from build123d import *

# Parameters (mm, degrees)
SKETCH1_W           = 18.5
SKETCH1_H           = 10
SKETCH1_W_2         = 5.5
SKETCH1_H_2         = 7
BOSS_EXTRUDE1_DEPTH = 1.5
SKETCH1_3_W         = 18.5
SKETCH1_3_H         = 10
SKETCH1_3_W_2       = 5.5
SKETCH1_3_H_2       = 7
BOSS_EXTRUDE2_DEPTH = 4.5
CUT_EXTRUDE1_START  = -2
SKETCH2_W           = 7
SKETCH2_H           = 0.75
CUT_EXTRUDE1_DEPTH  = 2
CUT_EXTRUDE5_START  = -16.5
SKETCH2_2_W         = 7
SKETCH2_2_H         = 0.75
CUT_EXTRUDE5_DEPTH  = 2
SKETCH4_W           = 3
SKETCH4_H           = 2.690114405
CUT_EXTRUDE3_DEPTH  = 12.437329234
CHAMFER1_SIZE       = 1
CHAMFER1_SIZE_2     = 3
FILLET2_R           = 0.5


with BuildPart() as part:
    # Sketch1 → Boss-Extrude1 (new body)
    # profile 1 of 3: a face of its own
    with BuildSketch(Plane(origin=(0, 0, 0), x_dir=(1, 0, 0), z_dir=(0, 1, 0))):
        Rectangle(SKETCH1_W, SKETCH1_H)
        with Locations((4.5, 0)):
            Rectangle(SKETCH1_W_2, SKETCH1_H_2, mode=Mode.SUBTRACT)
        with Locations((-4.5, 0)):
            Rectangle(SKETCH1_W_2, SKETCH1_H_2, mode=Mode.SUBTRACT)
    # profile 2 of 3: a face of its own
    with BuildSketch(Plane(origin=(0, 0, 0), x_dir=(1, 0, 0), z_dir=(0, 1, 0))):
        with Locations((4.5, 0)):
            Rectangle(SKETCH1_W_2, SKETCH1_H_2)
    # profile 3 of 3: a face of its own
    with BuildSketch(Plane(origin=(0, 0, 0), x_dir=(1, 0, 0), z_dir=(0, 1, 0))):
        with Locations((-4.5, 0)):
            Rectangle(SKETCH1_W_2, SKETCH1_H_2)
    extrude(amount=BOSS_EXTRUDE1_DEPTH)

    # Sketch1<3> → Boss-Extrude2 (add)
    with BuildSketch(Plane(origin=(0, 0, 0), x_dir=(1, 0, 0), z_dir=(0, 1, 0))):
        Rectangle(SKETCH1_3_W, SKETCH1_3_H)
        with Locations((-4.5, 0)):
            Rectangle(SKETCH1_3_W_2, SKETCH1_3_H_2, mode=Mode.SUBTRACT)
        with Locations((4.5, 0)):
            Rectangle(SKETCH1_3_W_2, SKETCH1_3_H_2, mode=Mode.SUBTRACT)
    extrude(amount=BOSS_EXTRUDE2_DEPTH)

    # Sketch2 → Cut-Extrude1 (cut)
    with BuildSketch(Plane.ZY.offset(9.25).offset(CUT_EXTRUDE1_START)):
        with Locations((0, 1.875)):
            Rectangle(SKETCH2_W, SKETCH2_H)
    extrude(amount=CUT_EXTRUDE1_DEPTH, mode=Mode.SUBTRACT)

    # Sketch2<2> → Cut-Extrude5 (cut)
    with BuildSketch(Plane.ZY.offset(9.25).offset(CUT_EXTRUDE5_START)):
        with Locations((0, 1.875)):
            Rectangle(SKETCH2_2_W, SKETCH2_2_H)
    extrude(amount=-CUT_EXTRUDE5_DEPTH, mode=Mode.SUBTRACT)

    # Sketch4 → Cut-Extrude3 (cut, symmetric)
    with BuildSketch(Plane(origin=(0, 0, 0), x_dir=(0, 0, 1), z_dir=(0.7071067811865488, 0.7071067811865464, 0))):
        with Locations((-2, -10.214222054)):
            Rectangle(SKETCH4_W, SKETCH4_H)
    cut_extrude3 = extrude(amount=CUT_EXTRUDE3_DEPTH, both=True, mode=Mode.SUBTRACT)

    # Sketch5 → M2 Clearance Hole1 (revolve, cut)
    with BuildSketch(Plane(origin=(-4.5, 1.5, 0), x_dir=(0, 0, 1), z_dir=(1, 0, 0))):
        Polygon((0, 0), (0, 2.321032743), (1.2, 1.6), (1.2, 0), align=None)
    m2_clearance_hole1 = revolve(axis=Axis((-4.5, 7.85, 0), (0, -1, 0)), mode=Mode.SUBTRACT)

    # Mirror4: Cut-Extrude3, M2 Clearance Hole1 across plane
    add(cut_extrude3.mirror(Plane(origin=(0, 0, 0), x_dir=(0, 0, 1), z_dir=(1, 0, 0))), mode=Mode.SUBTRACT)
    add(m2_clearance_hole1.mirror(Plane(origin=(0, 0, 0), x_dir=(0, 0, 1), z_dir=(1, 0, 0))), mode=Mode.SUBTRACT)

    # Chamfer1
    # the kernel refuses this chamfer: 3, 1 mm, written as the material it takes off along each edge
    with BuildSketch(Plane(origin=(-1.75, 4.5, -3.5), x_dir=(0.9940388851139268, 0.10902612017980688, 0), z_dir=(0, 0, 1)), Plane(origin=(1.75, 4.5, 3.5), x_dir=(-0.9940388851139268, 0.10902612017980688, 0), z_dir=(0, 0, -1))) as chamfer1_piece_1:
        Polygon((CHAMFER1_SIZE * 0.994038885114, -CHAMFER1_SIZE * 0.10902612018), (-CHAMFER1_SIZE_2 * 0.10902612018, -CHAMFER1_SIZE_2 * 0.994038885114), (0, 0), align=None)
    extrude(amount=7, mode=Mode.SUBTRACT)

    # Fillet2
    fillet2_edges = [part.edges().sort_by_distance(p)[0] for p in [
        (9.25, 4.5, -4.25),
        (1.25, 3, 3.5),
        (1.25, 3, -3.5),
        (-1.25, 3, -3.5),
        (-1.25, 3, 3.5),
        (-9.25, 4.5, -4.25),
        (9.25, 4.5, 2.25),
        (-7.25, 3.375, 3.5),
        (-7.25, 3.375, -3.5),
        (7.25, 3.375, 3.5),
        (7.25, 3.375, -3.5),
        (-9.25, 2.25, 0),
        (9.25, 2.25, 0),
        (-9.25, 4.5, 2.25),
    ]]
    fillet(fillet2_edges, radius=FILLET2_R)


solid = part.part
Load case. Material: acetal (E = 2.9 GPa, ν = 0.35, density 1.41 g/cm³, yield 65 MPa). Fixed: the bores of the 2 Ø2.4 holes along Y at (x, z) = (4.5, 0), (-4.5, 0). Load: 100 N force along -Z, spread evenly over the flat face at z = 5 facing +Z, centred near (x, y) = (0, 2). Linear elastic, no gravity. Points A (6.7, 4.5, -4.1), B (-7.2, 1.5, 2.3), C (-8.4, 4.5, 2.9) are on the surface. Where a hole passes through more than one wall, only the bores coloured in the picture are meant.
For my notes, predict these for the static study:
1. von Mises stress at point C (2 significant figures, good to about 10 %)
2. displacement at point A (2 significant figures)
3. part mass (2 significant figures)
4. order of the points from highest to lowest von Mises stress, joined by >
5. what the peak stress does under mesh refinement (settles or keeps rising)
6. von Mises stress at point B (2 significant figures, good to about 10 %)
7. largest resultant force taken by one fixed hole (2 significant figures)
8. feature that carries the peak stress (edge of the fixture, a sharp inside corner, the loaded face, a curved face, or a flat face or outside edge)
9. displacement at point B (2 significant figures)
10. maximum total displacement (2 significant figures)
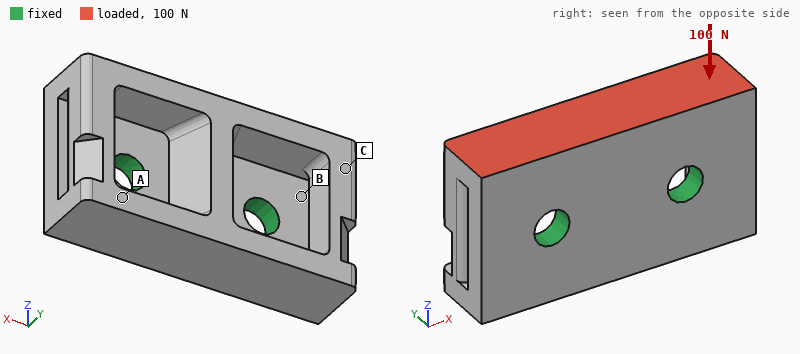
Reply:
4.9 MPa
48 µm
0.76 g
B > C > A
keeps rising
7.9 MPa
50 N
edge of the fixture
16 µm
71 µm
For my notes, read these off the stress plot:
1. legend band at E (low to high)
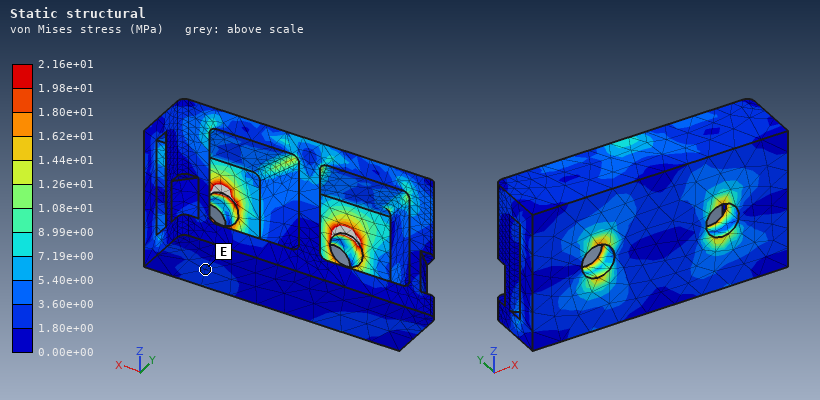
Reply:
1.80e+00 to 3.60e+00 MPa
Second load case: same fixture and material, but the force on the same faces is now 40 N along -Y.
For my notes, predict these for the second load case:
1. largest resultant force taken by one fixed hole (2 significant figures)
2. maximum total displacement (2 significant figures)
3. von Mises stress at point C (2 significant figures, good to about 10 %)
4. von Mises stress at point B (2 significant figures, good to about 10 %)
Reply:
20 N
70 µm
2.5 MPa
4.7 MPa
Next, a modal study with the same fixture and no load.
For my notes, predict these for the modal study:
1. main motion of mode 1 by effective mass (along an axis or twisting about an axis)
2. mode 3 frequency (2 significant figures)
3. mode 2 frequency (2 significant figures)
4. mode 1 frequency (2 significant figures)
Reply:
along Z
11 kHz
9900 Hz
7600 Hz
